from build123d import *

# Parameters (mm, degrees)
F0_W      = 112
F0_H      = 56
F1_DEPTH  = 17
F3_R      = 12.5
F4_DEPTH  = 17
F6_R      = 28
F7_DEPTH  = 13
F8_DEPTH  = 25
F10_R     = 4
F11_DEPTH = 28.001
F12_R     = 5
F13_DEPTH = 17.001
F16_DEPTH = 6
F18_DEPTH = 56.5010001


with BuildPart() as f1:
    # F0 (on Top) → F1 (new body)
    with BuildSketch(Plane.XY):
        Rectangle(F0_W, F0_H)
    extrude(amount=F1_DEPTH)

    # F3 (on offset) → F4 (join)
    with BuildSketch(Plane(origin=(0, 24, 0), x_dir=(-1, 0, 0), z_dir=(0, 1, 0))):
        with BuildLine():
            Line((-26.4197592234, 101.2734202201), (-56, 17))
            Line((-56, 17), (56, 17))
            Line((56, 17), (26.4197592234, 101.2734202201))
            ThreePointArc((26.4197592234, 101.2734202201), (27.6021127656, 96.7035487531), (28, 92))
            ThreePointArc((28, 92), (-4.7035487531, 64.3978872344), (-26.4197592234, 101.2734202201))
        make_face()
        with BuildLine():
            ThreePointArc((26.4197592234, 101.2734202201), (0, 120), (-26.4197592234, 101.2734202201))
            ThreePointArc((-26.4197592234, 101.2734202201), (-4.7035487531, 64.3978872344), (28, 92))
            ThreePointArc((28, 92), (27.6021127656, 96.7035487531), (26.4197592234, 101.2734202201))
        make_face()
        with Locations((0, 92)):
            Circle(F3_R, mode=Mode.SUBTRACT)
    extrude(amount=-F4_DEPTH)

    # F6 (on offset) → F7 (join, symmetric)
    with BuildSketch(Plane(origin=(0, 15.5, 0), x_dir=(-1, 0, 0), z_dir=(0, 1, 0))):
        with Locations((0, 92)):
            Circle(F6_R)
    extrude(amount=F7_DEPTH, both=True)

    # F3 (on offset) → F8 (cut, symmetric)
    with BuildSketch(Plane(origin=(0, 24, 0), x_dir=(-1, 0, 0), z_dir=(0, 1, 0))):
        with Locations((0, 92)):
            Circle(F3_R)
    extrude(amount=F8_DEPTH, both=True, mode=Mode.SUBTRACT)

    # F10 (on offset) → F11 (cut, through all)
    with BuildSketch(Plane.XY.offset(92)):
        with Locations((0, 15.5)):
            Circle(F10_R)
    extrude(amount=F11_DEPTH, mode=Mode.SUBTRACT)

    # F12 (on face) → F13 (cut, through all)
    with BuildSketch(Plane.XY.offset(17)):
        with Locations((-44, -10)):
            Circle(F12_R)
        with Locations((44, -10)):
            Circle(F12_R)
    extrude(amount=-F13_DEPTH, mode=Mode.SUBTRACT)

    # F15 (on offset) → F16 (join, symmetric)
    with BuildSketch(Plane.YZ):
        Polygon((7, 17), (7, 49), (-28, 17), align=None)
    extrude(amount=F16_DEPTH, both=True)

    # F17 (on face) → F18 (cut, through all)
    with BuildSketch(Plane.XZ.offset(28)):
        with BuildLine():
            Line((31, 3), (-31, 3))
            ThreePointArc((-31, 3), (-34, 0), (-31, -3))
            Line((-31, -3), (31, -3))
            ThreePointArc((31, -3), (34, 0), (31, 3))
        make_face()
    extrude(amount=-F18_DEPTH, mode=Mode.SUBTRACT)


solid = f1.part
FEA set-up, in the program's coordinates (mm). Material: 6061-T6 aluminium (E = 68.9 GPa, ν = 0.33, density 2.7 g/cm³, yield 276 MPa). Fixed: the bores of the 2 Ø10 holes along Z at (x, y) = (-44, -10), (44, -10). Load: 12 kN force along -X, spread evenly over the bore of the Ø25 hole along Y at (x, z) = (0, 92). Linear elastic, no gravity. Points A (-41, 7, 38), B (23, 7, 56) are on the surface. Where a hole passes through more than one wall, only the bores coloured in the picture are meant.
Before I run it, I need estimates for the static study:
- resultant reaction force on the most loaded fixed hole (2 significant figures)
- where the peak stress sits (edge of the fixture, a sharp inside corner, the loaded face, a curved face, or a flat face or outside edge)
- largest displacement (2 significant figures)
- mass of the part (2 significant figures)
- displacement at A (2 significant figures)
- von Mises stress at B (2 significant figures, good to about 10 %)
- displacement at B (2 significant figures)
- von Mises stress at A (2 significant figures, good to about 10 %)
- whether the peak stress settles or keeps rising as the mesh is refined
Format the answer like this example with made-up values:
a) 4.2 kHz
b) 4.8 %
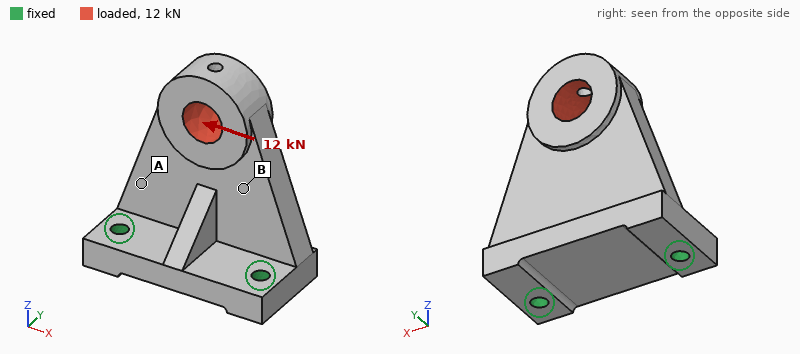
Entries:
a) 13 kN
b) edge of the fixture
c) 0.19 mm
d) 640 g
e) 0.069 mm
f) 22 MPa
g) 0.083 mm
h) 43 MPa
i) keeps rising
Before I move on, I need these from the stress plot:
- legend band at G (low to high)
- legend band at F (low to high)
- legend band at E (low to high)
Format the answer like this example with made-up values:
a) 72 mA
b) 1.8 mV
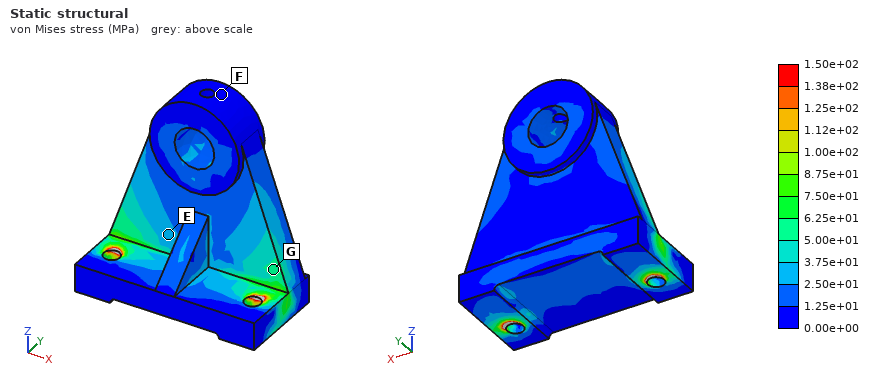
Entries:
a) 5.00e+01 to 6.25e+01 MPa
b) 0.00e+00 to 1.25e+01 MPa
c) 2.50e+01 to 3.75e+01 MPa
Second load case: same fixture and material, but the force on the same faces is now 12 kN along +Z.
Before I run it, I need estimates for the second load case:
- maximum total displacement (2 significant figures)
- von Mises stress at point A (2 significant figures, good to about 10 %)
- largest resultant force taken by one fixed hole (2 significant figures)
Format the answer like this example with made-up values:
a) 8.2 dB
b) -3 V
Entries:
a) 0.22 mm
b) 14 MPa
c) 6.1 kN
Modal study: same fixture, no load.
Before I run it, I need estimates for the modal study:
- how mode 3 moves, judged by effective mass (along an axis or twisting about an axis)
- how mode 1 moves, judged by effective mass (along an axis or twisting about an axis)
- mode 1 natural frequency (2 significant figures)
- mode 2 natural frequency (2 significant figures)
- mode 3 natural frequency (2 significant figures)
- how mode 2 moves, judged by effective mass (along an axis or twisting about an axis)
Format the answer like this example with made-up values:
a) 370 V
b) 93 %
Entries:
a) along Z
b) along Y
c) 1100 Hz
d) 3100 Hz
e) 4200 Hz
f) along X
